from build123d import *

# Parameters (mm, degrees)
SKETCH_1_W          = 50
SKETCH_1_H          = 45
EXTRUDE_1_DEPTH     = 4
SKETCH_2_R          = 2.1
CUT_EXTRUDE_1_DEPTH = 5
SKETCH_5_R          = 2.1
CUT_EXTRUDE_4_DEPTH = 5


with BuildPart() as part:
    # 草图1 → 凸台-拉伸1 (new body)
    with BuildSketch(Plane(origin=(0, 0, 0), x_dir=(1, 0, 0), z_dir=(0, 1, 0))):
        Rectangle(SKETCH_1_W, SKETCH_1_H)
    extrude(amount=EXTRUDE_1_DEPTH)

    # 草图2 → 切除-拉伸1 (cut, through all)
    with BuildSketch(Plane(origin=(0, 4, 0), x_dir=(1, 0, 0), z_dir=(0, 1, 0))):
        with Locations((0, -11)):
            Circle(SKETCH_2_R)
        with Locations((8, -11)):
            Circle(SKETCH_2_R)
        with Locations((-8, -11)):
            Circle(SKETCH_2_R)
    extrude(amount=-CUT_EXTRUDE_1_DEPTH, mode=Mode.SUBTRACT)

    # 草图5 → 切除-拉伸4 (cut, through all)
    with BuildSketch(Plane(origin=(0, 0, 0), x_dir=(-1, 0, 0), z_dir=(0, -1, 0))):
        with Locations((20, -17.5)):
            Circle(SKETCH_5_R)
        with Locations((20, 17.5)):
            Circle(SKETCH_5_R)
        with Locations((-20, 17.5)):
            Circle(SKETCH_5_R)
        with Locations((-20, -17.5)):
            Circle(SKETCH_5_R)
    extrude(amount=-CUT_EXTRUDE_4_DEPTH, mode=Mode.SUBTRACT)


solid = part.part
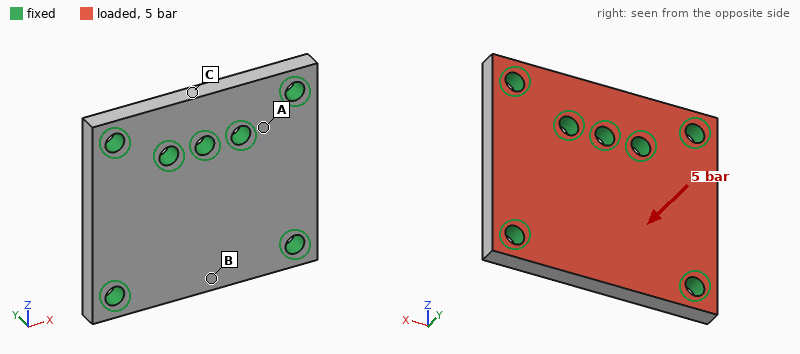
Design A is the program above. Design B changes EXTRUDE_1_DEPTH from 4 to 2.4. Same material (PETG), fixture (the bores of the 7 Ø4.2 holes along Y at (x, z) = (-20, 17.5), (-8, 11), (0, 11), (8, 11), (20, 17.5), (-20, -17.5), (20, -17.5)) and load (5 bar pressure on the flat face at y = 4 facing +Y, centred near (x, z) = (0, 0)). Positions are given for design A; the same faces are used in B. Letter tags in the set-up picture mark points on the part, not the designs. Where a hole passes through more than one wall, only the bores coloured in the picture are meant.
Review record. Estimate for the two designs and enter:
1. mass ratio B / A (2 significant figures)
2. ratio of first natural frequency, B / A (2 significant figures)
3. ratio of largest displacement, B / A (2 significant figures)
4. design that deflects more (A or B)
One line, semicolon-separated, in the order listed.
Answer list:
0.60; 0.65; 4.0; B
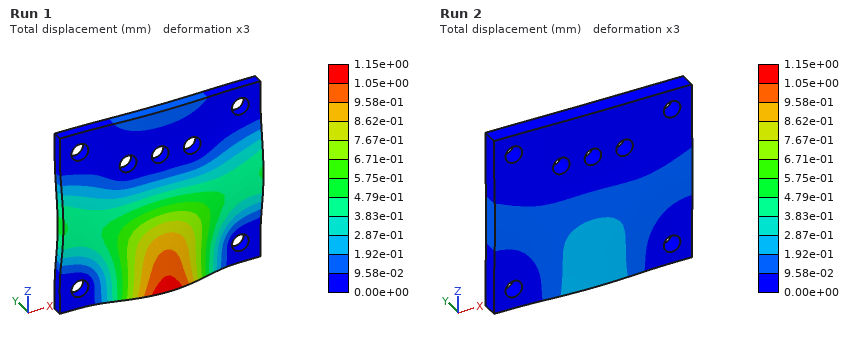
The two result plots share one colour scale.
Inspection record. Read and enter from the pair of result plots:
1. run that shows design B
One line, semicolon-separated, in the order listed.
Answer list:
Run 1
